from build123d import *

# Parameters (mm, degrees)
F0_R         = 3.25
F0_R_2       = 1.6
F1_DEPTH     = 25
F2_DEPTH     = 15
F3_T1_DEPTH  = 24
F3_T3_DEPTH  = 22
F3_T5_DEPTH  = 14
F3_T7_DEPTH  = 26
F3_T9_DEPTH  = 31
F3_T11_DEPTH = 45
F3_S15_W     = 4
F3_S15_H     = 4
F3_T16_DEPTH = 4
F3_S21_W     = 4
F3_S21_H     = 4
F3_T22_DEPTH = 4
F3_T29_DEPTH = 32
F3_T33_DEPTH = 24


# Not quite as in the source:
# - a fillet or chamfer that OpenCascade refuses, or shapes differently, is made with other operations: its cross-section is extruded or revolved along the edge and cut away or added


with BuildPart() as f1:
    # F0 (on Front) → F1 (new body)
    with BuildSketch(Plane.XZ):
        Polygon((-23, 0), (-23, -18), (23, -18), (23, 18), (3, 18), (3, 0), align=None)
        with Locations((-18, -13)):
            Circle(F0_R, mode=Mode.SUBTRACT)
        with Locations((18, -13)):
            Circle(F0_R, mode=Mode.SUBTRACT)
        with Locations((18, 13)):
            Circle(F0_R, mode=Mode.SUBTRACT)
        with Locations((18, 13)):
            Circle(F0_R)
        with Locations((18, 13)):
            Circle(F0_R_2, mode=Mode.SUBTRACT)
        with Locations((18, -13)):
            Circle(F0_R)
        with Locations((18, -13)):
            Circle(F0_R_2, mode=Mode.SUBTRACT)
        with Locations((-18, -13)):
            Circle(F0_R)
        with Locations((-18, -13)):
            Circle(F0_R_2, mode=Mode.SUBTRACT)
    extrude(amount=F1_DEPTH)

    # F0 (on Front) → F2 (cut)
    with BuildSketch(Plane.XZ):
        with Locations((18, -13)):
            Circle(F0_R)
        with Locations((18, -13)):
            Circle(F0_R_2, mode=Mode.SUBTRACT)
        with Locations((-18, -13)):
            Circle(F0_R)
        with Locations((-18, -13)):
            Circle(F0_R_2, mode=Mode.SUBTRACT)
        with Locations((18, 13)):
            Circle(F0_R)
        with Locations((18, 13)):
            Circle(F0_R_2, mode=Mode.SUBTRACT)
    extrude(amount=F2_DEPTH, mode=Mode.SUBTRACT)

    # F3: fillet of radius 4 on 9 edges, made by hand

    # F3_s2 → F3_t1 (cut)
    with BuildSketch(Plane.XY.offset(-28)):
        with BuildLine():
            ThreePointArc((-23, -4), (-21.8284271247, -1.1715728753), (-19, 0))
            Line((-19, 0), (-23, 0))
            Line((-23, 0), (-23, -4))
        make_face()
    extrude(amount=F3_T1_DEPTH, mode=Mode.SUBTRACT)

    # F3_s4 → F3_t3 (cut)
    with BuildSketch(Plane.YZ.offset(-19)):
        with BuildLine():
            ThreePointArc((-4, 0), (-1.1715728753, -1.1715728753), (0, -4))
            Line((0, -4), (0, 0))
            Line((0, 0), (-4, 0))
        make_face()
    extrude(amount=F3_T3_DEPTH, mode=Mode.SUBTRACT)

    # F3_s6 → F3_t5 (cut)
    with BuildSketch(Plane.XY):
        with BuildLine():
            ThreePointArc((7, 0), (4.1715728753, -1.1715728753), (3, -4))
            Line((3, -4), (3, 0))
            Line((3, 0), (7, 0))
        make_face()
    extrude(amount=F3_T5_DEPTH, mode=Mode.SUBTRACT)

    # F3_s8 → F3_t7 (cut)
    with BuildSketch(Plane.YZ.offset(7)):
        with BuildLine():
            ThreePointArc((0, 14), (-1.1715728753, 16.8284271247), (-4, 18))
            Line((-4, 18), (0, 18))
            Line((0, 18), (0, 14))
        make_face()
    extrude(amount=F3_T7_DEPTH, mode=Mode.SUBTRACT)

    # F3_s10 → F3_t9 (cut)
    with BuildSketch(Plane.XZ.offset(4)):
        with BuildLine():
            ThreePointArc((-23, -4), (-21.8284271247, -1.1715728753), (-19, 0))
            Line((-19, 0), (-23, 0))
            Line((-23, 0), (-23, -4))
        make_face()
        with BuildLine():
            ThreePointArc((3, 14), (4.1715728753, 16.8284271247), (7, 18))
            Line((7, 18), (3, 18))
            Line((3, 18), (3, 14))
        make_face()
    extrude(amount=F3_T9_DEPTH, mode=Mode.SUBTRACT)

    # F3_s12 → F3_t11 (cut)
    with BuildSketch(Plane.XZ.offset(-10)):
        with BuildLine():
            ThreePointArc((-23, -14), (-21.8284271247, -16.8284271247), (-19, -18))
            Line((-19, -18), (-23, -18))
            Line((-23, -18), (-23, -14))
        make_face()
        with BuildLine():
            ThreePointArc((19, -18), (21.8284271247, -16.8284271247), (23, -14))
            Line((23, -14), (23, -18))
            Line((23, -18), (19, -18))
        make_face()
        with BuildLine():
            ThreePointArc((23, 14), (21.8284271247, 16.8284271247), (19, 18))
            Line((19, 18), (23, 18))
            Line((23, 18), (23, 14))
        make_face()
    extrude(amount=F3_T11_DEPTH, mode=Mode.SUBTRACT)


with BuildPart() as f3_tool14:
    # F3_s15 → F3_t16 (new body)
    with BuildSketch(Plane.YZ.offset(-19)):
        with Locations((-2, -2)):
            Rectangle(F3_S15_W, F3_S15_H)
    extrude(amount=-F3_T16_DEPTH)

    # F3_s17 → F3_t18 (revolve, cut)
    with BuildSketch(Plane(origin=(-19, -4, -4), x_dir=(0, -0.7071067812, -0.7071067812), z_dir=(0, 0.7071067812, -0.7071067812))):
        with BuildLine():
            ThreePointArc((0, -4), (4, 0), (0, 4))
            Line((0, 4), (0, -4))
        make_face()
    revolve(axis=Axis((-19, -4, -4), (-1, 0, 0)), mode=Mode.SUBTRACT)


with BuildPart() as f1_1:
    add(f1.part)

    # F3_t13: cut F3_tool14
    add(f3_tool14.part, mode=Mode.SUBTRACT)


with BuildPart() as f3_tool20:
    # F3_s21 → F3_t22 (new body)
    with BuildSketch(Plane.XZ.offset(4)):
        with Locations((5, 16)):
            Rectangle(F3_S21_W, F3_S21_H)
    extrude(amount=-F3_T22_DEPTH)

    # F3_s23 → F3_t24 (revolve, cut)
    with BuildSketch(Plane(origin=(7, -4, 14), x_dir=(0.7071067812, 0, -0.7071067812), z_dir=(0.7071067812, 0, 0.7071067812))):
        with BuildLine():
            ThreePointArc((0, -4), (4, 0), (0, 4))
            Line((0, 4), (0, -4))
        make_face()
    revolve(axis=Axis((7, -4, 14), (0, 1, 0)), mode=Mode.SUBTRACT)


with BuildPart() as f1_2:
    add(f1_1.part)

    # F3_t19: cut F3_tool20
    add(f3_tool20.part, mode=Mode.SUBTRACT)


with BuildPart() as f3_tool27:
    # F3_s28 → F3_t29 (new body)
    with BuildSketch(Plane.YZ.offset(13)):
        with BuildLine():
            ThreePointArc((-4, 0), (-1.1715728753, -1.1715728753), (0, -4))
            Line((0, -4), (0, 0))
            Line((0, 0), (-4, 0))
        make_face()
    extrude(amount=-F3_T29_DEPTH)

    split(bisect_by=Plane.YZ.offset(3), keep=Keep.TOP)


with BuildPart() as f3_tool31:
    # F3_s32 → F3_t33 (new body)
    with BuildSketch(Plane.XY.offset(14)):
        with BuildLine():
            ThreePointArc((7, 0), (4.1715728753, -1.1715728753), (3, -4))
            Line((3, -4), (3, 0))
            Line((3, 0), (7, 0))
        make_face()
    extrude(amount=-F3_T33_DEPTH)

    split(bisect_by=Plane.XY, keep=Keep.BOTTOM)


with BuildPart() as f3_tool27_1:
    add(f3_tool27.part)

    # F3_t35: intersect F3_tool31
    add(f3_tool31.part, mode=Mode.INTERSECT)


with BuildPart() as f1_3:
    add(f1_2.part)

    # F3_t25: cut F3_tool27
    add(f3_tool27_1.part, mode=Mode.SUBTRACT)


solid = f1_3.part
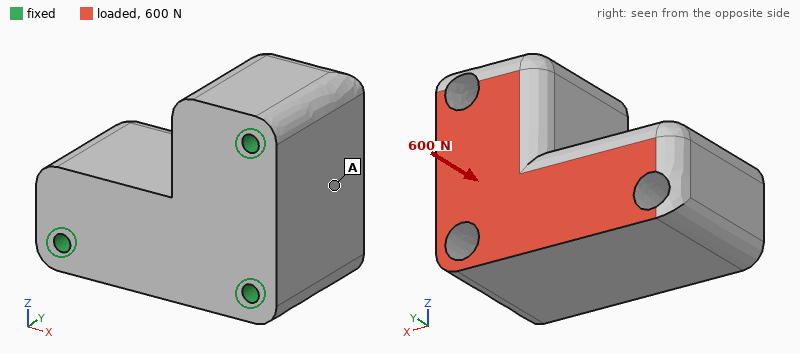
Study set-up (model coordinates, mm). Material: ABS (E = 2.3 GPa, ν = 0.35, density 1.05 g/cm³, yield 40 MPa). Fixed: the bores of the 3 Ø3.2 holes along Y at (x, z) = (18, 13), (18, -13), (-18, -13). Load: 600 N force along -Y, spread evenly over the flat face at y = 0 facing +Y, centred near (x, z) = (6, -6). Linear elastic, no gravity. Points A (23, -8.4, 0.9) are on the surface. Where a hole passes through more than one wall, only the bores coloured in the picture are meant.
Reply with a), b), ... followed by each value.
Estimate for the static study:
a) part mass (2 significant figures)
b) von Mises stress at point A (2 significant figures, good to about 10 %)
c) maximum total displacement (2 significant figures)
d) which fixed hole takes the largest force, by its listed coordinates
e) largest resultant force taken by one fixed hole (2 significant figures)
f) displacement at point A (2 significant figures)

a) 29 g
b) 0.61 MPa
c) 19 µm
d) (18, -13)
e) 250 N
f) 11 µm
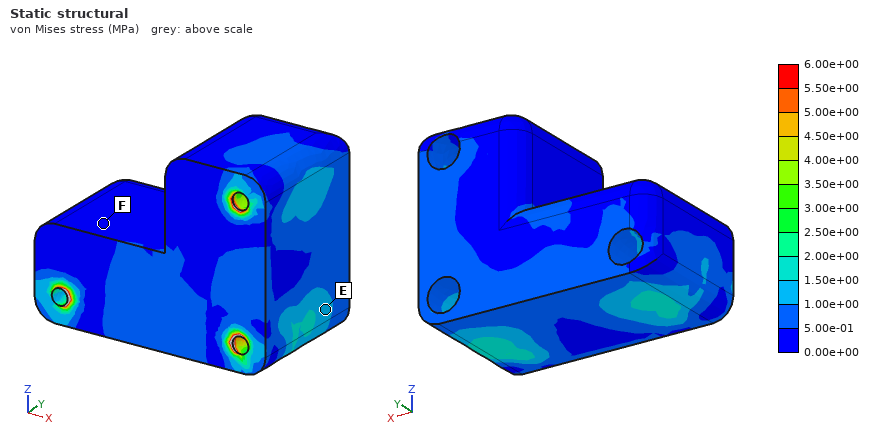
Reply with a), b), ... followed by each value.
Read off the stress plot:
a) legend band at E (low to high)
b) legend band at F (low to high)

a) 1.00e+00 to 1.50e+00 MPa
b) 0.00e+00 to 5.00e-01 MPa
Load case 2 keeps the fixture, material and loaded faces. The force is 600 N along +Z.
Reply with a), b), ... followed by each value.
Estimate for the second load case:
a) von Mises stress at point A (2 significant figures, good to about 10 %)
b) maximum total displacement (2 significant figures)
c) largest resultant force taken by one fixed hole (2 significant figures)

a) 2.5 MPa
b) 81 µm
c) 460 N
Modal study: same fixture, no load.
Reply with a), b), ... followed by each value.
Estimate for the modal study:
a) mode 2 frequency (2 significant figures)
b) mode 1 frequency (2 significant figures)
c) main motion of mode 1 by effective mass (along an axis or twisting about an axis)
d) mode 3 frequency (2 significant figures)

a) 6200 Hz
b) 4800 Hz
c) along Z
d) 6900 Hz
